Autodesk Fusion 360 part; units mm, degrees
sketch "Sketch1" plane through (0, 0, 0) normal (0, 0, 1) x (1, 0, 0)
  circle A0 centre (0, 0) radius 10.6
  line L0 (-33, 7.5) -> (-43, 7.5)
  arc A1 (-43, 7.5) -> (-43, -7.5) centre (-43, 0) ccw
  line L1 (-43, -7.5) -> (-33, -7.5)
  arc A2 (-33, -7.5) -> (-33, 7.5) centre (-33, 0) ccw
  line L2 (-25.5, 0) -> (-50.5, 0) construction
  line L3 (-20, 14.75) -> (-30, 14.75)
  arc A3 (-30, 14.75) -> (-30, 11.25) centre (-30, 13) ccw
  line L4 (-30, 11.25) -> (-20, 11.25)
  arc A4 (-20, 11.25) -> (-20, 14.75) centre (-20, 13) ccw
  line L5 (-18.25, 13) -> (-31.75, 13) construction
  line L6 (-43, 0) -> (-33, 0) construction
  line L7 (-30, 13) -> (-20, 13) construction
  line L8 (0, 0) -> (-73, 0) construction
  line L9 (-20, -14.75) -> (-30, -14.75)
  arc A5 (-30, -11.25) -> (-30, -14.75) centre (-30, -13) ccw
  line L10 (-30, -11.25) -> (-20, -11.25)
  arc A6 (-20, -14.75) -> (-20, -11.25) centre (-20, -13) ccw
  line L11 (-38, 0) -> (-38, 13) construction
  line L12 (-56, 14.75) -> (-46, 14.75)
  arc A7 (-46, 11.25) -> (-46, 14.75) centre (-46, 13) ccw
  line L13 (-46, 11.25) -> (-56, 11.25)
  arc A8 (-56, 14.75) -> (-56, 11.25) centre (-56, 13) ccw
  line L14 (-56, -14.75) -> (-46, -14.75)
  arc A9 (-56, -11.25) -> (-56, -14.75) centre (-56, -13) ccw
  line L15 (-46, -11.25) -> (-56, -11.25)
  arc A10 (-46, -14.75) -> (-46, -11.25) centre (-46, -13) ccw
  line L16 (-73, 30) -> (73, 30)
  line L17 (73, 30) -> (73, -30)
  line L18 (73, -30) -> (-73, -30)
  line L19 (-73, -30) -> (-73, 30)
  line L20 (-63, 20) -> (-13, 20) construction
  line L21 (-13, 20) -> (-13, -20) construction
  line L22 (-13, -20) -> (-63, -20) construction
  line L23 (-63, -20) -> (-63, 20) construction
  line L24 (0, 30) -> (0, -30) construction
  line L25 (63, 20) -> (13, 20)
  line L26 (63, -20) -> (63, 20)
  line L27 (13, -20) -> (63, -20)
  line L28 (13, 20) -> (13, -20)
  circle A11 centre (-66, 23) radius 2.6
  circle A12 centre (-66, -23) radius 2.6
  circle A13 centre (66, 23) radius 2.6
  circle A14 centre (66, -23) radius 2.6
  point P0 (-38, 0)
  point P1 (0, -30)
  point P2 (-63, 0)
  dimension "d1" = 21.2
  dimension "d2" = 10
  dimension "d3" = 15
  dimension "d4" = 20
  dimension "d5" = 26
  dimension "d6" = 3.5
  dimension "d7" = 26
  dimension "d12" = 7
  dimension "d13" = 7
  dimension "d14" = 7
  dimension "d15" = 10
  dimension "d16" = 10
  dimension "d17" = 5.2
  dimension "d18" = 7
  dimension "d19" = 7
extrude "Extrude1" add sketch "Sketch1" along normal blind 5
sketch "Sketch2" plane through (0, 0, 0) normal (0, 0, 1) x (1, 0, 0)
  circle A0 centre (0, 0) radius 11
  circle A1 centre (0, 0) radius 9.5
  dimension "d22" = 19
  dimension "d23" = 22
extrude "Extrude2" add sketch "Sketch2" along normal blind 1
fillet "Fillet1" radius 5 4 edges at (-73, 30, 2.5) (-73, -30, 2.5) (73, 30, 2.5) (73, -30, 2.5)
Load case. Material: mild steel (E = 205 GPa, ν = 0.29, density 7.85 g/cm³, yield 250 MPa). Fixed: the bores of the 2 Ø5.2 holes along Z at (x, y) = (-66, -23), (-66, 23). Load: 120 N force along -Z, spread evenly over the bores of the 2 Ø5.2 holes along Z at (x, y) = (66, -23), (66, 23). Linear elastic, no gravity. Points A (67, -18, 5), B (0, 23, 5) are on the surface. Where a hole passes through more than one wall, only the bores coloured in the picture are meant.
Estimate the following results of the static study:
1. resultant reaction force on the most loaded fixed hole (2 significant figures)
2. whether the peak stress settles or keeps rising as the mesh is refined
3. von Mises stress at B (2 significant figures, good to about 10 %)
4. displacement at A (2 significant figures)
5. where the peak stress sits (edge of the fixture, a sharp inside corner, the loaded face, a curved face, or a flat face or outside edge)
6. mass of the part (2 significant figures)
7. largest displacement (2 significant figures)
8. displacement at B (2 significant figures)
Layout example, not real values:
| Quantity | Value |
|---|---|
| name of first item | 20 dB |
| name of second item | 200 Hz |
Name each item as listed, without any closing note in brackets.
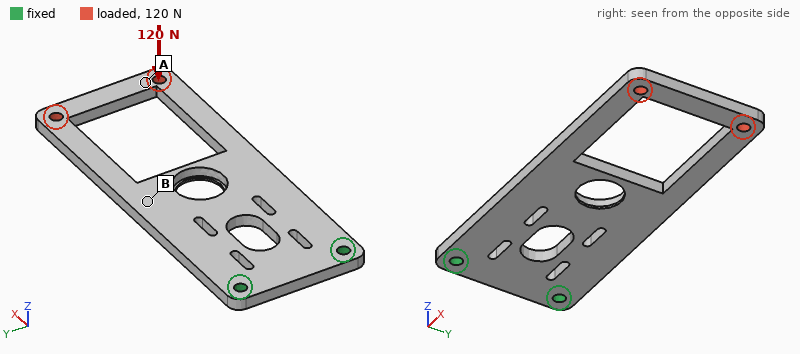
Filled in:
| Quantity | Value |
|---|---|
| resultant reaction force on the most loaded fixed hole | 60 N |
| whether the peak stress settles or keeps rising as the mesh is refined | keeps rising |
| von Mises stress at B | 48 MPa |
| displacement at A | 1.1 mm |
| where the peak stress sits | edge of the fixture |
| mass of the part | 230 g |
| largest displacement | 1.2 mm |
| displacement at B | 0.31 mm |
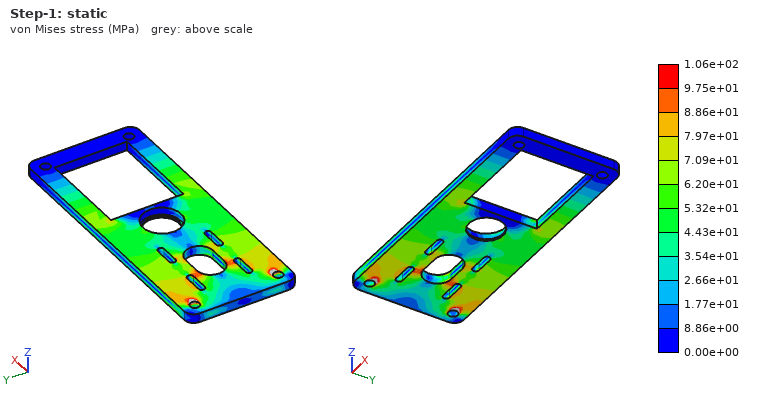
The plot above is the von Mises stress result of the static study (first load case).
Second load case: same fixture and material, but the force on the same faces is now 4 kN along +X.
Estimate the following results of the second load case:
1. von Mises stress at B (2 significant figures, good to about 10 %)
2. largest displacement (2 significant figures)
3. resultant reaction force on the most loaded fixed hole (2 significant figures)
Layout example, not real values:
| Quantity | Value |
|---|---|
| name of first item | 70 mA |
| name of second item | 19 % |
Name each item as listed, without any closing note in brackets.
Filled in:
| Quantity | Value |
|---|---|
| von Mises stress at B | 26 MPa |
| largest displacement | 27 µm |
| resultant reaction force on the most loaded fixed hole | 2.0 kN |
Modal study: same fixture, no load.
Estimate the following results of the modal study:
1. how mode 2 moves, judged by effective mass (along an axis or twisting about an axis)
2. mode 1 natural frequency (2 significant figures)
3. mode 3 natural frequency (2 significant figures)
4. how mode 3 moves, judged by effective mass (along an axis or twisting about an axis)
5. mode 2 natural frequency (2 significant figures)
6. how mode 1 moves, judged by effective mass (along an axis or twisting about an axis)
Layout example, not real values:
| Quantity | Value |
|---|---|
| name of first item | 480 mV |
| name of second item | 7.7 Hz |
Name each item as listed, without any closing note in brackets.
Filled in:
| Quantity | Value |
|---|---|
| how mode 2 moves, judged by effective mass | twisting about X |
| mode 1 natural frequency | 250 Hz |
| mode 3 natural frequency | 1100 Hz |
| how mode 3 moves, judged by effective mass | along Z |
| mode 2 natural frequency | 890 Hz |
| how mode 1 moves, judged by effective mass | along Z |
